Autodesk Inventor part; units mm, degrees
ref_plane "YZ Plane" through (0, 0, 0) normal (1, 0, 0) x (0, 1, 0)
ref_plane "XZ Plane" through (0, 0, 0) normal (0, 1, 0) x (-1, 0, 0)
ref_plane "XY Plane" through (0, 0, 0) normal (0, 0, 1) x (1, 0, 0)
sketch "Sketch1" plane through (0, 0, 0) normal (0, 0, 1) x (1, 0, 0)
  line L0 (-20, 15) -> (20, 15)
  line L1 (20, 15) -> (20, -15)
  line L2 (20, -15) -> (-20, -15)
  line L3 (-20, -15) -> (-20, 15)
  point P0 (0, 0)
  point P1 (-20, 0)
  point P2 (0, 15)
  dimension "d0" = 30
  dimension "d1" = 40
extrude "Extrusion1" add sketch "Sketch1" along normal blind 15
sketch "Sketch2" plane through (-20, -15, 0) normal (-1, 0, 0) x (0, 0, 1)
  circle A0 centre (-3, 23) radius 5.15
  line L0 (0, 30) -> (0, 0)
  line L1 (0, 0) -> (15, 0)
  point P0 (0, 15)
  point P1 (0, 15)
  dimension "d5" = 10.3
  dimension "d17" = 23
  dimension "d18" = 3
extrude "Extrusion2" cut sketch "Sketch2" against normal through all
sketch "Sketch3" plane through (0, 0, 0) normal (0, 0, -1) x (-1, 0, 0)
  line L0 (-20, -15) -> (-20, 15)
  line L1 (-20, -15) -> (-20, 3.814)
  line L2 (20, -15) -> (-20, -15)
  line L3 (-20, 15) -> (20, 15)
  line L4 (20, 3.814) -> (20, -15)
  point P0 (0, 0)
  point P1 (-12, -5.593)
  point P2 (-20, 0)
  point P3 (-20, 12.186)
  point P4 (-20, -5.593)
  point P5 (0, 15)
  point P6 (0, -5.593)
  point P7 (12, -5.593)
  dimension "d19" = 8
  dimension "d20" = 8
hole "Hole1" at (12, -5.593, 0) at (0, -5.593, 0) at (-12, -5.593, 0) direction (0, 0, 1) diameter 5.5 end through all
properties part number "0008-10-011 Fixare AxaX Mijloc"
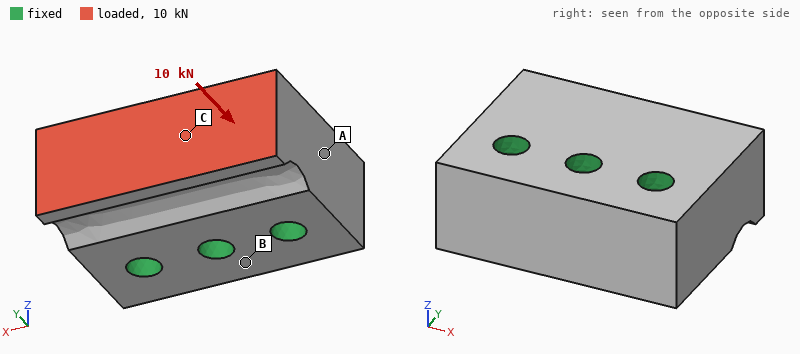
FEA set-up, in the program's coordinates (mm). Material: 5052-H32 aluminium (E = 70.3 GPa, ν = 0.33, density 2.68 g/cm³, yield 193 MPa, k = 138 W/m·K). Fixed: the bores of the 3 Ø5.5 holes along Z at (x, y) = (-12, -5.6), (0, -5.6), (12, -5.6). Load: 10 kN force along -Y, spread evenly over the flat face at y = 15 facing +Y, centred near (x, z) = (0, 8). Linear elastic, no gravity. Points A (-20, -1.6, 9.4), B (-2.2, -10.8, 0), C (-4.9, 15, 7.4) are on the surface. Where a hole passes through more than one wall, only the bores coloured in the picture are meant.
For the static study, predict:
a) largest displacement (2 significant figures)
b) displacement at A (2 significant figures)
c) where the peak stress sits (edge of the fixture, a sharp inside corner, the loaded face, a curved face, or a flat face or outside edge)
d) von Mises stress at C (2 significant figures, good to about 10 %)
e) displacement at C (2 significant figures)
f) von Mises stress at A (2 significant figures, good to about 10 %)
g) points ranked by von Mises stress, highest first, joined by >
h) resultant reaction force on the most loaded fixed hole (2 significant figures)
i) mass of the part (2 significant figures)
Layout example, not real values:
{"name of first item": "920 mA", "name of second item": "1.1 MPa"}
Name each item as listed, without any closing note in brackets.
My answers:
{"largest displacement": "8.3 µm", "displacement at A": "2.2 µm", "where the peak stress sits": "a curved face", "von Mises stress at C": "22 MPa", "displacement at C": "4.9 µm", "von Mises stress at A": "11 MPa", "points ranked by von Mises stress, highest first, joined by >": "C > A > B", "resultant reaction force on the most loaded fixed hole": "3.7 kN", "mass of the part": "44 g"}
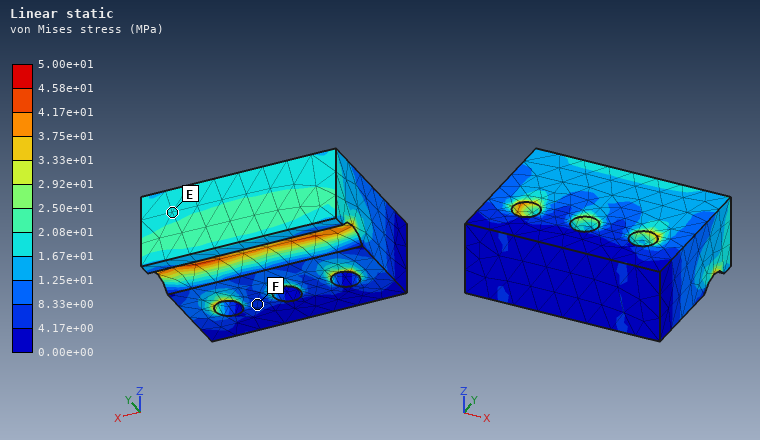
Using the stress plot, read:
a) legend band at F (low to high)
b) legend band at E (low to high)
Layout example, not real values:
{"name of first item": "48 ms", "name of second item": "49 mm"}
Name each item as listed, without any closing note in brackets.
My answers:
{"legend band at F": "4.17e+00 to 8.33e+00 MPa", "legend band at E": "1.67e+01 to 2.08e+01 MPa"}
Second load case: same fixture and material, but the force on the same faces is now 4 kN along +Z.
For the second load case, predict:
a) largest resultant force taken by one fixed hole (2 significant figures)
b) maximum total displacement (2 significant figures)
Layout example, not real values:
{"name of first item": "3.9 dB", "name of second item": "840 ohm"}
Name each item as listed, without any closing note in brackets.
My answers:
{"largest resultant force taken by one fixed hole": "1.4 kN", "maximum total displacement": "23 µm"}
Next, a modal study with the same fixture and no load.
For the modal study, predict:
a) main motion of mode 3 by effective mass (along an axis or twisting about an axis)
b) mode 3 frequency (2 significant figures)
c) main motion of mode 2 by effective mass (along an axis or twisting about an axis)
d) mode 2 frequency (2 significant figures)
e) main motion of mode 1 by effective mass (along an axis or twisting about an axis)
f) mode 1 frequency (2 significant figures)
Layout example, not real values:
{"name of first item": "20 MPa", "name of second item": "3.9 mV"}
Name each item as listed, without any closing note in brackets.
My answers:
{"main motion of mode 3 by effective mass": "along X", "mode 3 frequency": "32 kHz", "main motion of mode 2 by effective mass": "twisting about Y", "mode 2 frequency": "30 kHz", "main motion of mode 1 by effective mass": "along Z", "mode 1 frequency": "25 kHz"}
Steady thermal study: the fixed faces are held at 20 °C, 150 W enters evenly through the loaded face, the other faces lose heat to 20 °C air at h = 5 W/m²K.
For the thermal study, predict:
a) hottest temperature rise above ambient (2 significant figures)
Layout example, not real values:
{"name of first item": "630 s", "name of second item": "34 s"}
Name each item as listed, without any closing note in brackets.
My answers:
{"hottest temperature rise above ambient": "39 K"}
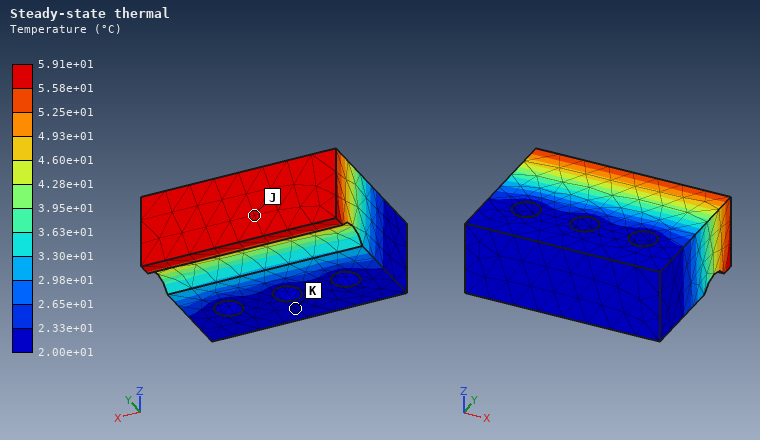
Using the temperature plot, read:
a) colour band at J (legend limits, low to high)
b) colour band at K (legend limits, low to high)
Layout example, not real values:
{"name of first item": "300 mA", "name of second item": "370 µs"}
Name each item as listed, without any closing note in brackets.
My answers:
{"colour band at J": "5.58e+01 to 5.91e+01 °C", "colour band at K": "2.00e+01 to 2.33e+01 °C"}
